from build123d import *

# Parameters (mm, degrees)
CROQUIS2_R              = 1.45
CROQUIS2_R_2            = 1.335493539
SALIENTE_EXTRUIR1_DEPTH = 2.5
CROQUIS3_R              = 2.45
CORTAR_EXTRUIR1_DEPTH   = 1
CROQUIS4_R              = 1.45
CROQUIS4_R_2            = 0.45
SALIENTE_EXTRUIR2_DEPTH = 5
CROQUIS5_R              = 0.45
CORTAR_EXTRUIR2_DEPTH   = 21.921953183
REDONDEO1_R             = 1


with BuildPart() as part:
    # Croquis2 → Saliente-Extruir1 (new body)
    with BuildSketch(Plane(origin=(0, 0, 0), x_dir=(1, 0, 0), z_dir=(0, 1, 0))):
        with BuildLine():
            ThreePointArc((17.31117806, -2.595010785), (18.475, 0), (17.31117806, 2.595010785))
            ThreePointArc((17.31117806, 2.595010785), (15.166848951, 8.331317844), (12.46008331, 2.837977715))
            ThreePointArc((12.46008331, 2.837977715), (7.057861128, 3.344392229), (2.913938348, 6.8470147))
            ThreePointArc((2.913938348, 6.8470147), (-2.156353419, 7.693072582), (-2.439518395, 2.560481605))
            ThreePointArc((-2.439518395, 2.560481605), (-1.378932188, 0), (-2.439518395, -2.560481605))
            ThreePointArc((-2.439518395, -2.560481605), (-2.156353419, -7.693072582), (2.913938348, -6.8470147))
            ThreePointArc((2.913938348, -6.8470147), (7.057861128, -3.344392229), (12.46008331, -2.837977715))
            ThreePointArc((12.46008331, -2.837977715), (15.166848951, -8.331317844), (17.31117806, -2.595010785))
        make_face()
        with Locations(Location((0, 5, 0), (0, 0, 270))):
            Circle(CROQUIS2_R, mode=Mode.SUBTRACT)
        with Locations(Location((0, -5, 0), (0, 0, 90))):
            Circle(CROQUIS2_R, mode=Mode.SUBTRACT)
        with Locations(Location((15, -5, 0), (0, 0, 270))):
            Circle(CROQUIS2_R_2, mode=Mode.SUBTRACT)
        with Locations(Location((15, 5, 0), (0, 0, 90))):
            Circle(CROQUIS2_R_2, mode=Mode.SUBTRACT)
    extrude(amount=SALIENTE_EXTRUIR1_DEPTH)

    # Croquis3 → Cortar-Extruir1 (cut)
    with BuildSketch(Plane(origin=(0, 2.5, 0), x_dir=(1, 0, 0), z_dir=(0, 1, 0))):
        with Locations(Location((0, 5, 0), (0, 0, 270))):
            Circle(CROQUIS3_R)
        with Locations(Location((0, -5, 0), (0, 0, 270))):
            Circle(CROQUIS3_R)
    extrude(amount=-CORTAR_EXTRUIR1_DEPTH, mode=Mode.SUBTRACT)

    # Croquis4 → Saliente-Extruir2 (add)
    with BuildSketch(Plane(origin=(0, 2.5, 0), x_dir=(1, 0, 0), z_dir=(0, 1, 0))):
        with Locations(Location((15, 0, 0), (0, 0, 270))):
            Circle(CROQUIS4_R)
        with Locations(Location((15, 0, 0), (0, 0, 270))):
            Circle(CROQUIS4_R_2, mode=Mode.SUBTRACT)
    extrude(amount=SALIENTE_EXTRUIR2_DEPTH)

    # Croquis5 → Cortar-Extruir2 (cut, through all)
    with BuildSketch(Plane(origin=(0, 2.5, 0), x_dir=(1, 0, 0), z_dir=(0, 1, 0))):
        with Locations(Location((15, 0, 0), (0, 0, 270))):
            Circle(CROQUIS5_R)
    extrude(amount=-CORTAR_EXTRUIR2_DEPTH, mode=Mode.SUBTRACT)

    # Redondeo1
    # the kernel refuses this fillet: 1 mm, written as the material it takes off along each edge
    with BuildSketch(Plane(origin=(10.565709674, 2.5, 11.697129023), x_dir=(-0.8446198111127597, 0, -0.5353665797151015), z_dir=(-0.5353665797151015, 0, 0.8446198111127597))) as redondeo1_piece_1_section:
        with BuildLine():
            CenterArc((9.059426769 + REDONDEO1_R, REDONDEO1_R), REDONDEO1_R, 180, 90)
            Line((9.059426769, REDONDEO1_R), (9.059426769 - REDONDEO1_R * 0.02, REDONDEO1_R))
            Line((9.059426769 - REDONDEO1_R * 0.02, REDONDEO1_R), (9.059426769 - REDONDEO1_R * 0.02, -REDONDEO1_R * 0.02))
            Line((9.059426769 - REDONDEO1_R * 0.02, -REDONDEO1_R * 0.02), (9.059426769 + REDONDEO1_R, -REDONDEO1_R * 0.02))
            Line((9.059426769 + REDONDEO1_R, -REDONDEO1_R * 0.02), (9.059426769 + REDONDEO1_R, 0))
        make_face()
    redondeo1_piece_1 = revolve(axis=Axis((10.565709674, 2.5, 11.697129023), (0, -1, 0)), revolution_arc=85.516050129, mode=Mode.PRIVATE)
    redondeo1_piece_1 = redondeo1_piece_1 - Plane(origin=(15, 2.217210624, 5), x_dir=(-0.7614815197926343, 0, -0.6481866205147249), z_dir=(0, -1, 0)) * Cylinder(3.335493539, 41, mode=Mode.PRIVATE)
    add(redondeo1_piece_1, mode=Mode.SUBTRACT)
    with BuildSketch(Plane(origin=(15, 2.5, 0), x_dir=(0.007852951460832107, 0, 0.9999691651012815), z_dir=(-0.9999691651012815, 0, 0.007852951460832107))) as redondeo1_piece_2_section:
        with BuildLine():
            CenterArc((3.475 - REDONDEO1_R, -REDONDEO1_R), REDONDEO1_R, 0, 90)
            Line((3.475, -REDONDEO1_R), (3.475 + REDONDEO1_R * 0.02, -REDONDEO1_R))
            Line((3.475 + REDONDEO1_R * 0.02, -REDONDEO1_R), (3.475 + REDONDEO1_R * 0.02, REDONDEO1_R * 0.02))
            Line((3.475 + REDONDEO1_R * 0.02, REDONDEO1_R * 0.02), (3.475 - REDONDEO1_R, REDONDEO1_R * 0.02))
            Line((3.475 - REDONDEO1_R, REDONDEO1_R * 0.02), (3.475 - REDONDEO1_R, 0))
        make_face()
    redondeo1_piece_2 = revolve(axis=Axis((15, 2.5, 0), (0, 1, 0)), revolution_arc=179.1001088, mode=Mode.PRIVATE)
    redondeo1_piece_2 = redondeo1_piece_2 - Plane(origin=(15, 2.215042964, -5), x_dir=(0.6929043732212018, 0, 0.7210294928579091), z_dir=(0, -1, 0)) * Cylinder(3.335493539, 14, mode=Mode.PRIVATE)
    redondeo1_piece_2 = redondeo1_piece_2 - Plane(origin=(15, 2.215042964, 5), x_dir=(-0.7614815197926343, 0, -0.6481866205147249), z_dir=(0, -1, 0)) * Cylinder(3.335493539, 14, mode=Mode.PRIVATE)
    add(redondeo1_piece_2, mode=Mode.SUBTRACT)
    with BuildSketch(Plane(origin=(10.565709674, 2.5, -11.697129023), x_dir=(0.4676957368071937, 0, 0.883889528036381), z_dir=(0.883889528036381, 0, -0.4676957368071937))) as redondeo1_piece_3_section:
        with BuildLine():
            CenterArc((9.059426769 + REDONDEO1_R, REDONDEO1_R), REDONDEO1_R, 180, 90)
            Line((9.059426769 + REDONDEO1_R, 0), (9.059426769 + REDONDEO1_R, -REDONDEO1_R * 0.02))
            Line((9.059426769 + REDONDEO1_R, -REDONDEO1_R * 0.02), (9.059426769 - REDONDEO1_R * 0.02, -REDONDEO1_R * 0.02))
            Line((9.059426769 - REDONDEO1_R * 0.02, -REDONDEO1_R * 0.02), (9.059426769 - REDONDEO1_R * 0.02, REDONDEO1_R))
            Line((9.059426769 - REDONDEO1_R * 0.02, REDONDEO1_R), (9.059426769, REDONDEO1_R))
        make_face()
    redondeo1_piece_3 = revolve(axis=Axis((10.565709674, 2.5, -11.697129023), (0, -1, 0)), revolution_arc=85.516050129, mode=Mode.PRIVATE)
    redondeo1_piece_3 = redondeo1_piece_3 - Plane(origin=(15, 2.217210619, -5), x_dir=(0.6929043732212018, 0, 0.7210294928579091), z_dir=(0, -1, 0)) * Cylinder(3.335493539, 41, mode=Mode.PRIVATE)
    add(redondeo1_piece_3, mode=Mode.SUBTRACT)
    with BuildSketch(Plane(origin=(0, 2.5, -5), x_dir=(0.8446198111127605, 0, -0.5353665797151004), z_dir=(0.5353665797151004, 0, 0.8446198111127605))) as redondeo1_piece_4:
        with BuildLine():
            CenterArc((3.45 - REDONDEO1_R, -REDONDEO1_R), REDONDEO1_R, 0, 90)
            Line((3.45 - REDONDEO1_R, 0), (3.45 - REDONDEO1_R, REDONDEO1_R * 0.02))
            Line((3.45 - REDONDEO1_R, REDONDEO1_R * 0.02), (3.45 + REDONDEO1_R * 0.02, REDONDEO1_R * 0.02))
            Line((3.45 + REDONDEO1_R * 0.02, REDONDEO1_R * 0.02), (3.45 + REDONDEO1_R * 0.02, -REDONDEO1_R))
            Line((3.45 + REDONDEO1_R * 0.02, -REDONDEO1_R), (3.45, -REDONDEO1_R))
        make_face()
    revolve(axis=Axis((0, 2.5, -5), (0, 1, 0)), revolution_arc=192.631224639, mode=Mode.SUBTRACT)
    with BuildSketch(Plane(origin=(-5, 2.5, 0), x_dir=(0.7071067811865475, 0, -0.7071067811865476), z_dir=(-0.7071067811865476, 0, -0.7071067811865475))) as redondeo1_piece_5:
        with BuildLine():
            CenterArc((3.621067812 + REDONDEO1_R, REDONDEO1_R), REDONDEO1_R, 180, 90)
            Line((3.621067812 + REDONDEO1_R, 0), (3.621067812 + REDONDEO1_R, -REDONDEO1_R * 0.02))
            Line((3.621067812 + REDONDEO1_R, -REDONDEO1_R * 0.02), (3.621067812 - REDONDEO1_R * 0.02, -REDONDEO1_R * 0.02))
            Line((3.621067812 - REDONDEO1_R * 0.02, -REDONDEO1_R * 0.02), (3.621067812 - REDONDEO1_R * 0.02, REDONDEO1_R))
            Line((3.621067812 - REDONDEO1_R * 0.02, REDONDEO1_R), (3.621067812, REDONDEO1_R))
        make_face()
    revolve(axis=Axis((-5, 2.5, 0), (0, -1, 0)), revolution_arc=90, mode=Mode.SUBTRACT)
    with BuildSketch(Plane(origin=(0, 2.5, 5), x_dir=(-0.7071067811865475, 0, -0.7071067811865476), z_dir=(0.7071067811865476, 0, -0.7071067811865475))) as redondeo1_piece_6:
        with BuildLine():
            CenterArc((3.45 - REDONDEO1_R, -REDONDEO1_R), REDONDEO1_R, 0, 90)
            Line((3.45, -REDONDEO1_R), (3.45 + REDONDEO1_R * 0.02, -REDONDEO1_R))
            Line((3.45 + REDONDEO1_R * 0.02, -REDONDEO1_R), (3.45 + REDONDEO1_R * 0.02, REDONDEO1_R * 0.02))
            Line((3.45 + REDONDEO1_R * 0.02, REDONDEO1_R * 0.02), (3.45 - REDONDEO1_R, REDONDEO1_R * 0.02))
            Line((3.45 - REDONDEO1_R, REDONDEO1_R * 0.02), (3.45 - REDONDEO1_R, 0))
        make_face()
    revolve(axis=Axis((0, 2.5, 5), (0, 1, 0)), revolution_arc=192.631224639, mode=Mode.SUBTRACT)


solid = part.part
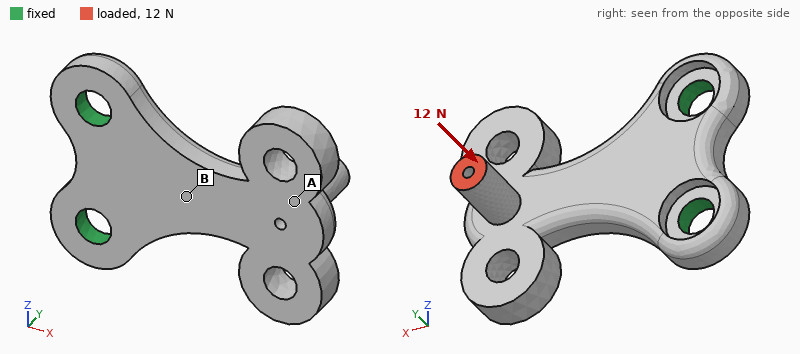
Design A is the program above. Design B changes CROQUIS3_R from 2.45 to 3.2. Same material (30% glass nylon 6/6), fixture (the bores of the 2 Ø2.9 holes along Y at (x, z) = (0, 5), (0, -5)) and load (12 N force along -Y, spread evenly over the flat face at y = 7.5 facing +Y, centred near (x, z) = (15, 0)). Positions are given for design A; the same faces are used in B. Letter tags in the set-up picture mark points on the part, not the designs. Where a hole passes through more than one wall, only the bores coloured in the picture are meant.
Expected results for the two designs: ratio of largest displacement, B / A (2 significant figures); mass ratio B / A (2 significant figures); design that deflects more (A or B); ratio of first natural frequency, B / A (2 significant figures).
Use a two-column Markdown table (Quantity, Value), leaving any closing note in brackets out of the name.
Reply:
| Quantity | Value |
|---|---|
| ratio of largest displacement, B / A | 1.1 |
| mass ratio B / A | 0.96 |
| design that deflects more | B |
| ratio of first natural frequency, B / A | 0.93 |
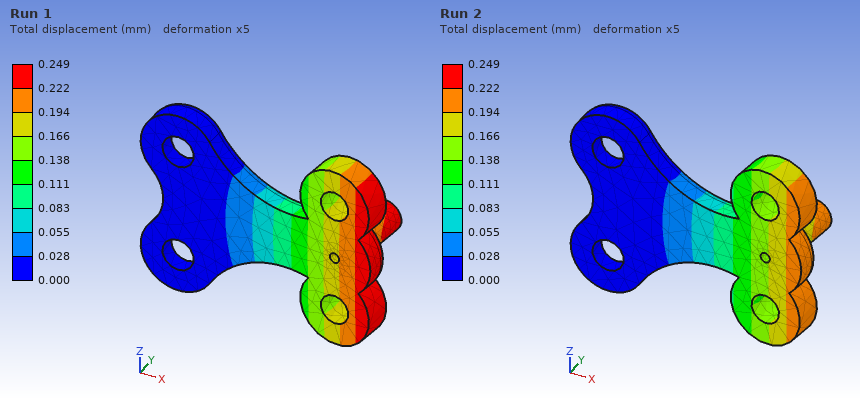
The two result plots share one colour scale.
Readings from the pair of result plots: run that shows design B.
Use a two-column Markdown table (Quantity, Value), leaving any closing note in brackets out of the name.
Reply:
| Quantity | Value |
|---|---|
| run that shows design B | Run 1 |
